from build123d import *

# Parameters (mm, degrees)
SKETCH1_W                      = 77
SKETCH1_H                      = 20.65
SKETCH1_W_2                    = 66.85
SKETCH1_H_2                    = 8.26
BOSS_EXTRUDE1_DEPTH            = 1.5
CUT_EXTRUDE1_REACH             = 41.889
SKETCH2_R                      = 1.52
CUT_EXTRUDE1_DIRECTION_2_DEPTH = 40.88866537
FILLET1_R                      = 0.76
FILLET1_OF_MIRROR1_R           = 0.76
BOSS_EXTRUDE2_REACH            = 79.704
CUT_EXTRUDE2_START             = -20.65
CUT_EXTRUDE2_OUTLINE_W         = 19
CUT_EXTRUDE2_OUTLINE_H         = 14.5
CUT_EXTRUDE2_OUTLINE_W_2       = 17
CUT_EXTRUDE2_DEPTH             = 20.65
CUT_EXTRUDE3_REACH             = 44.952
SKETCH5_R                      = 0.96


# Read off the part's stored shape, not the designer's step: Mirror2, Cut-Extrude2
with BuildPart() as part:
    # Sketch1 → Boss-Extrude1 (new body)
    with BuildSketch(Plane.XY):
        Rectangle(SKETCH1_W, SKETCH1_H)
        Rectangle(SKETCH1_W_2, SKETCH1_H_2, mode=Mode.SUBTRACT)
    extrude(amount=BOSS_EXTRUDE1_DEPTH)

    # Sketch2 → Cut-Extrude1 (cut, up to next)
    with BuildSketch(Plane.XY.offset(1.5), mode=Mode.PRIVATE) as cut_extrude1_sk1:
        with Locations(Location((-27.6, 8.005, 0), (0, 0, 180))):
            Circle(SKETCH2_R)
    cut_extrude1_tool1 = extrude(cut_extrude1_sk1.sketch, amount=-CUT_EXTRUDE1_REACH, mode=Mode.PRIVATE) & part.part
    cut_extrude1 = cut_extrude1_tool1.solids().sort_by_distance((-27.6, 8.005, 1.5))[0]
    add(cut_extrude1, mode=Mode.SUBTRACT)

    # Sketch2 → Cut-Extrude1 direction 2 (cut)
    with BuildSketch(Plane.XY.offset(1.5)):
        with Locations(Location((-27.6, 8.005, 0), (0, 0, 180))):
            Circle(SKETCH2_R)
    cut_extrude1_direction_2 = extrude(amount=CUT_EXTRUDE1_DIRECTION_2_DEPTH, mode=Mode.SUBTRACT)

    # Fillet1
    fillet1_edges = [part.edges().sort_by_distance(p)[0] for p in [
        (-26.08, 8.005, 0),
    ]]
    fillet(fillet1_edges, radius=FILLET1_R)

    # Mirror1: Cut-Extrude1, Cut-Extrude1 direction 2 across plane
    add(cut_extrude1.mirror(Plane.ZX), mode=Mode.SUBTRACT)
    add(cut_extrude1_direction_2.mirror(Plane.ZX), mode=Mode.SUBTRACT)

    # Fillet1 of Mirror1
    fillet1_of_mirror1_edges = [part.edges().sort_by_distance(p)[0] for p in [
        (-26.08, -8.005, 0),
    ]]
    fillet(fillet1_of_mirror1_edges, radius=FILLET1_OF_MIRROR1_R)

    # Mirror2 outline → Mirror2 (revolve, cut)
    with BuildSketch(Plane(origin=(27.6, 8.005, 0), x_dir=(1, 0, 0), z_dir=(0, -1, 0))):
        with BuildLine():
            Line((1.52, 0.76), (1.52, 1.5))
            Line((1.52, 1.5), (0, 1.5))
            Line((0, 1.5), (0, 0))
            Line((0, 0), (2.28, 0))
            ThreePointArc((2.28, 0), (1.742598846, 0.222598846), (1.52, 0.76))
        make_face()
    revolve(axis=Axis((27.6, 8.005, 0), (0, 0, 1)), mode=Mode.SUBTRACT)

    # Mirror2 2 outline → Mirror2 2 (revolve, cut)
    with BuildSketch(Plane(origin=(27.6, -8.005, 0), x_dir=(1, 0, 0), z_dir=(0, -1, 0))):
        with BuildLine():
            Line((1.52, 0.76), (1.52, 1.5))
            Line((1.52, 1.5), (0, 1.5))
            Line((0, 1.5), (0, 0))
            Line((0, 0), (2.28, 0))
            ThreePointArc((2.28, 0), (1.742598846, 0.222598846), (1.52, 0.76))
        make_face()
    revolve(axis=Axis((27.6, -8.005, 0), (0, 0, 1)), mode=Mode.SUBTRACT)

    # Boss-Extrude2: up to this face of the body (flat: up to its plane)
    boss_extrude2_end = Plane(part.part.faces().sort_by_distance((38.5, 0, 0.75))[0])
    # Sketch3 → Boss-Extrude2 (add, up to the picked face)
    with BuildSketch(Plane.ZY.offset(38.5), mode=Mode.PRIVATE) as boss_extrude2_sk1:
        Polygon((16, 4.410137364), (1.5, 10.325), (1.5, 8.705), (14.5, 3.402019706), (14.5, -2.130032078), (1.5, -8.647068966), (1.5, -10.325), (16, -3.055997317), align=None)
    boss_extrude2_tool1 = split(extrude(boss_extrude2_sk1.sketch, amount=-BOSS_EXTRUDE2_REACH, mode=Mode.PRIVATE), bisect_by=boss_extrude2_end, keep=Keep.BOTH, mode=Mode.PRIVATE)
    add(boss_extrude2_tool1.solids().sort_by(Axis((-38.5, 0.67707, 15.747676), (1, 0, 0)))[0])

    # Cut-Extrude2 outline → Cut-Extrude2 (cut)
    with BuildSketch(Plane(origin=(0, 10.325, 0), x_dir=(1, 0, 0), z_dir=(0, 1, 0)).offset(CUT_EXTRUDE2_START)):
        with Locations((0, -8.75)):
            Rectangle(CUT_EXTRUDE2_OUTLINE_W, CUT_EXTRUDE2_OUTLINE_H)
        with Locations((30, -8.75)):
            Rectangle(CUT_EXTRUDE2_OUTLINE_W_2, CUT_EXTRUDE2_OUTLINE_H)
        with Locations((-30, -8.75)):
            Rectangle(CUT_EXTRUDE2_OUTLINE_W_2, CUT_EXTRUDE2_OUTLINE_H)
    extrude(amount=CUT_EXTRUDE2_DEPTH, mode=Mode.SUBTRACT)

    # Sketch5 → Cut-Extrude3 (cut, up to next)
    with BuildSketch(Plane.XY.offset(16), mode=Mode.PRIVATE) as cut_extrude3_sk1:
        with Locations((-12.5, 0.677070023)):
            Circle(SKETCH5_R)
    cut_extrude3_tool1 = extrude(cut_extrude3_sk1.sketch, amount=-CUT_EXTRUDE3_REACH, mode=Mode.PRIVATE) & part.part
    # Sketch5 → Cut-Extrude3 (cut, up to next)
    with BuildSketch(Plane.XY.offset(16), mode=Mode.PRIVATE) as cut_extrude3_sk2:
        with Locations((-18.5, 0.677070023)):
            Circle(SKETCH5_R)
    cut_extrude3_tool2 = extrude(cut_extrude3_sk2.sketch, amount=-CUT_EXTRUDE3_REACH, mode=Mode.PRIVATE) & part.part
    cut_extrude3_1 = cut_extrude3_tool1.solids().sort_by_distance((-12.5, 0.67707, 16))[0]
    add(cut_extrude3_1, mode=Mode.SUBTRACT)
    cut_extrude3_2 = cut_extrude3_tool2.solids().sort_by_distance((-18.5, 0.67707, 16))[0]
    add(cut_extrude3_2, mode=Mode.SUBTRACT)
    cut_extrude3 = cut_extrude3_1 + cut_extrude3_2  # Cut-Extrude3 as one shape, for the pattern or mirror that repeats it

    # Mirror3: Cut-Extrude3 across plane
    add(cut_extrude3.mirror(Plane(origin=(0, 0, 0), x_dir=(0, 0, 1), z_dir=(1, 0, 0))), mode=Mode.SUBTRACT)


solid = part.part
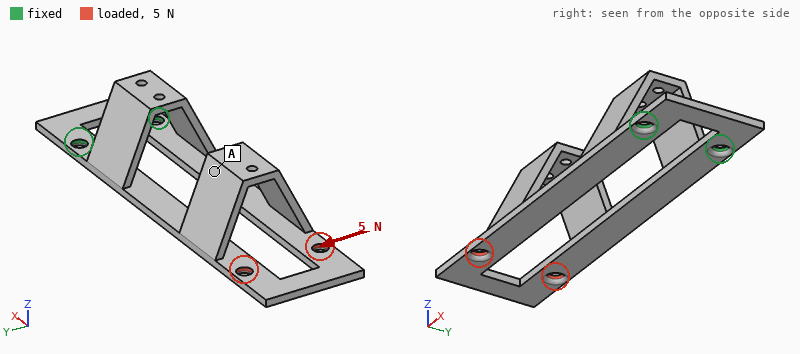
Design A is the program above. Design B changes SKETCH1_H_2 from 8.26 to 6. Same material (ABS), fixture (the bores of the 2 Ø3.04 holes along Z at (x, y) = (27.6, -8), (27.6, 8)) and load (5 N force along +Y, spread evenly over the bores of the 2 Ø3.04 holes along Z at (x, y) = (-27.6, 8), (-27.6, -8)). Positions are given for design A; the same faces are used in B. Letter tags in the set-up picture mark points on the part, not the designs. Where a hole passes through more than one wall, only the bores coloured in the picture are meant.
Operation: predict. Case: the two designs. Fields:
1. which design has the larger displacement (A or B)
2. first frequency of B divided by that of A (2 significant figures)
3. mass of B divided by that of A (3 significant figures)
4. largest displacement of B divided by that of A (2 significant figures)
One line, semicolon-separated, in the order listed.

A; 1.0; 1.08; 0.69
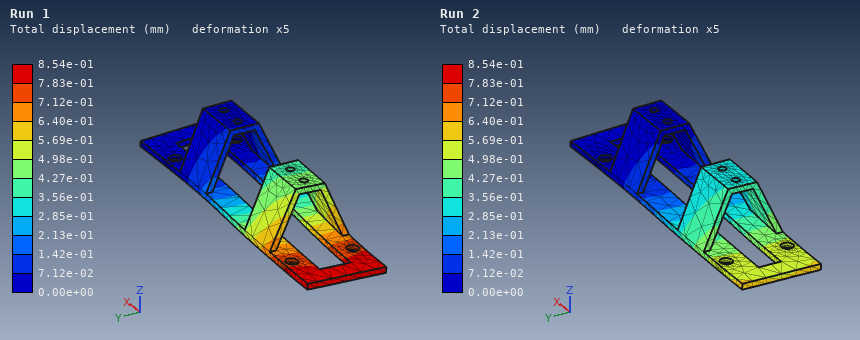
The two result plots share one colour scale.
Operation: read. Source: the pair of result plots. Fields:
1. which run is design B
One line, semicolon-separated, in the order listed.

Run 2
